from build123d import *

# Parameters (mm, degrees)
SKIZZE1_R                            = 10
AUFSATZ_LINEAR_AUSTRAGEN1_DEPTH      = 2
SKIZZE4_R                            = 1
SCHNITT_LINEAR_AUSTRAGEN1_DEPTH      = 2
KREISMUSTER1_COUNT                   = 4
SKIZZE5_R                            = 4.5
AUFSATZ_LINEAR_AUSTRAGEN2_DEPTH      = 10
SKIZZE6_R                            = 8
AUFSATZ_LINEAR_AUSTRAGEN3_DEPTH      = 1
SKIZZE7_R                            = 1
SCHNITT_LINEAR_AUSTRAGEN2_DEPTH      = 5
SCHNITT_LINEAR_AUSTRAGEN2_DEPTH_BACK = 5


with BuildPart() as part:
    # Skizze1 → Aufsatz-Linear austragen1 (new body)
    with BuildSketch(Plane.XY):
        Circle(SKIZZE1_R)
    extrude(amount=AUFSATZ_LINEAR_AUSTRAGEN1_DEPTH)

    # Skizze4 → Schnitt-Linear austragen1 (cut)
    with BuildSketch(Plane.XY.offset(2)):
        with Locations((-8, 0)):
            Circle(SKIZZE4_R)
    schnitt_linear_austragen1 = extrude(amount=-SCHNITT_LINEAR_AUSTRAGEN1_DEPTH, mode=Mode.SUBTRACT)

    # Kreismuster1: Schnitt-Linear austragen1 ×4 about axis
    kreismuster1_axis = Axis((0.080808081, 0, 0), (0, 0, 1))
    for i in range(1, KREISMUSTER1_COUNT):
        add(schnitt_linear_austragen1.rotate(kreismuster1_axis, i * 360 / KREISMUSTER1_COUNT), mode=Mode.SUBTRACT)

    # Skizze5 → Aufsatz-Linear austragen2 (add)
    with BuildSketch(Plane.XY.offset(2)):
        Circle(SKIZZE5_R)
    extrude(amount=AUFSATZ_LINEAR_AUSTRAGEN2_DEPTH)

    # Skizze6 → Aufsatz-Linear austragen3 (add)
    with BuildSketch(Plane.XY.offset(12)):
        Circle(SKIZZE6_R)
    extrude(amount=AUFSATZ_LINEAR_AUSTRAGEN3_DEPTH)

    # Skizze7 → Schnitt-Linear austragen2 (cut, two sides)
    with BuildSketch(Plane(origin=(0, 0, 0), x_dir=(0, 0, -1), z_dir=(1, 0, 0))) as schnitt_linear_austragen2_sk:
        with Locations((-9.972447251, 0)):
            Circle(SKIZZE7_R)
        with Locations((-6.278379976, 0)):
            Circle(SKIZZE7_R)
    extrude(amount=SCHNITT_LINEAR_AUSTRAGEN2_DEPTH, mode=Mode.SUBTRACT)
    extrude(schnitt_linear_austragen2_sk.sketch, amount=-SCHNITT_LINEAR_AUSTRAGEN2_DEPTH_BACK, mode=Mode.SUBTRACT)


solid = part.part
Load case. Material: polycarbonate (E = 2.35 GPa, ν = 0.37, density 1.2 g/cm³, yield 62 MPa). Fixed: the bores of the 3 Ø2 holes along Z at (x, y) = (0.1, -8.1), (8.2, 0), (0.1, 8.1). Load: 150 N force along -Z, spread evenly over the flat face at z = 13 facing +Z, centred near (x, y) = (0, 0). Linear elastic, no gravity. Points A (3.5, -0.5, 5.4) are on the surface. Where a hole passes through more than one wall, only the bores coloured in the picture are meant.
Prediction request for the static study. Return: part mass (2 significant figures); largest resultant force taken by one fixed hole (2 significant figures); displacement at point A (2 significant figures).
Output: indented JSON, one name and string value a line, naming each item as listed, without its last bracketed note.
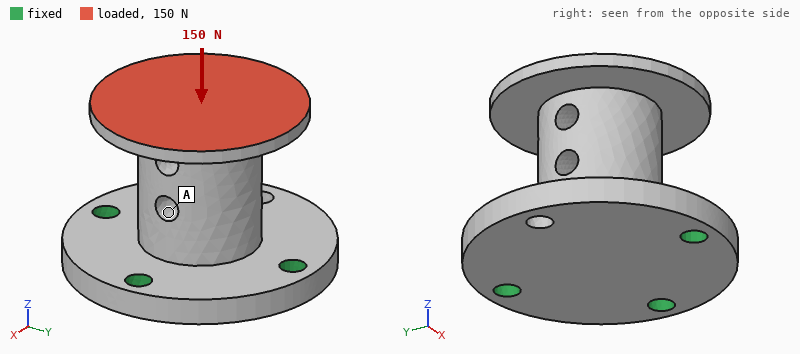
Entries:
{
  "part mass": "1.7 g",
  "largest resultant force taken by one fixed hole": "68 N",
  "displacement at point A": "0.054 mm"
}
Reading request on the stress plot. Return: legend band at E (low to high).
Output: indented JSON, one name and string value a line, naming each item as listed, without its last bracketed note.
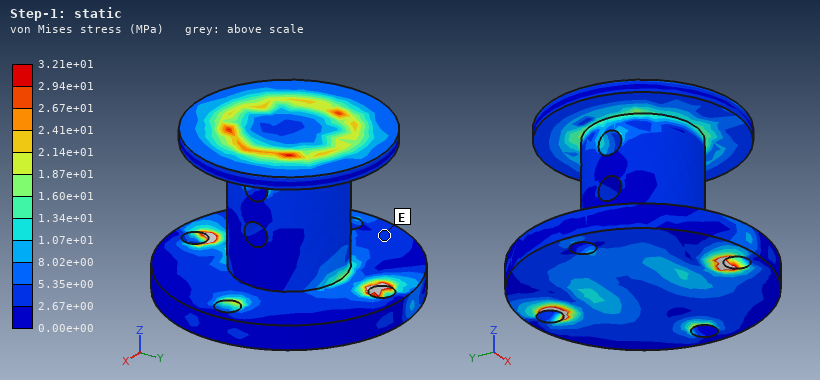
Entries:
{
  "legend band at E": "2.67e+00 to 5.35e+00 MPa"
}
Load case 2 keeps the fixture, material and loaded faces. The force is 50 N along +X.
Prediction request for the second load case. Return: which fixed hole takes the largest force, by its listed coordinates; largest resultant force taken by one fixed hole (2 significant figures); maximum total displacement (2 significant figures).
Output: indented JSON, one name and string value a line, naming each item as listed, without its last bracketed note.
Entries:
{
  "which fixed hole takes the largest force, by its listed coordinates": "(8.2, 0)",
  "largest resultant force taken by one fixed hole": "69 N",
  "maximum total displacement": "0.36 mm"
}
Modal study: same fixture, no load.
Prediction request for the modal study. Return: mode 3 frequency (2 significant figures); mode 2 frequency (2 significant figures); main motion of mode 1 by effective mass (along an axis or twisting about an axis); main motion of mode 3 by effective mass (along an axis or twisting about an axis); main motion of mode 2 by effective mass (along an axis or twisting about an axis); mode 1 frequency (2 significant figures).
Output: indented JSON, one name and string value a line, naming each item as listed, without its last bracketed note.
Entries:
{
  "mode 3 frequency": "7200 Hz",
  "mode 2 frequency": "4500 Hz",
  "main motion of mode 1 by effective mass": "along X",
  "main motion of mode 3 by effective mass": "along Z",
  "main motion of mode 2 by effective mass": "along Y",
  "mode 1 frequency": "2900 Hz"
}
